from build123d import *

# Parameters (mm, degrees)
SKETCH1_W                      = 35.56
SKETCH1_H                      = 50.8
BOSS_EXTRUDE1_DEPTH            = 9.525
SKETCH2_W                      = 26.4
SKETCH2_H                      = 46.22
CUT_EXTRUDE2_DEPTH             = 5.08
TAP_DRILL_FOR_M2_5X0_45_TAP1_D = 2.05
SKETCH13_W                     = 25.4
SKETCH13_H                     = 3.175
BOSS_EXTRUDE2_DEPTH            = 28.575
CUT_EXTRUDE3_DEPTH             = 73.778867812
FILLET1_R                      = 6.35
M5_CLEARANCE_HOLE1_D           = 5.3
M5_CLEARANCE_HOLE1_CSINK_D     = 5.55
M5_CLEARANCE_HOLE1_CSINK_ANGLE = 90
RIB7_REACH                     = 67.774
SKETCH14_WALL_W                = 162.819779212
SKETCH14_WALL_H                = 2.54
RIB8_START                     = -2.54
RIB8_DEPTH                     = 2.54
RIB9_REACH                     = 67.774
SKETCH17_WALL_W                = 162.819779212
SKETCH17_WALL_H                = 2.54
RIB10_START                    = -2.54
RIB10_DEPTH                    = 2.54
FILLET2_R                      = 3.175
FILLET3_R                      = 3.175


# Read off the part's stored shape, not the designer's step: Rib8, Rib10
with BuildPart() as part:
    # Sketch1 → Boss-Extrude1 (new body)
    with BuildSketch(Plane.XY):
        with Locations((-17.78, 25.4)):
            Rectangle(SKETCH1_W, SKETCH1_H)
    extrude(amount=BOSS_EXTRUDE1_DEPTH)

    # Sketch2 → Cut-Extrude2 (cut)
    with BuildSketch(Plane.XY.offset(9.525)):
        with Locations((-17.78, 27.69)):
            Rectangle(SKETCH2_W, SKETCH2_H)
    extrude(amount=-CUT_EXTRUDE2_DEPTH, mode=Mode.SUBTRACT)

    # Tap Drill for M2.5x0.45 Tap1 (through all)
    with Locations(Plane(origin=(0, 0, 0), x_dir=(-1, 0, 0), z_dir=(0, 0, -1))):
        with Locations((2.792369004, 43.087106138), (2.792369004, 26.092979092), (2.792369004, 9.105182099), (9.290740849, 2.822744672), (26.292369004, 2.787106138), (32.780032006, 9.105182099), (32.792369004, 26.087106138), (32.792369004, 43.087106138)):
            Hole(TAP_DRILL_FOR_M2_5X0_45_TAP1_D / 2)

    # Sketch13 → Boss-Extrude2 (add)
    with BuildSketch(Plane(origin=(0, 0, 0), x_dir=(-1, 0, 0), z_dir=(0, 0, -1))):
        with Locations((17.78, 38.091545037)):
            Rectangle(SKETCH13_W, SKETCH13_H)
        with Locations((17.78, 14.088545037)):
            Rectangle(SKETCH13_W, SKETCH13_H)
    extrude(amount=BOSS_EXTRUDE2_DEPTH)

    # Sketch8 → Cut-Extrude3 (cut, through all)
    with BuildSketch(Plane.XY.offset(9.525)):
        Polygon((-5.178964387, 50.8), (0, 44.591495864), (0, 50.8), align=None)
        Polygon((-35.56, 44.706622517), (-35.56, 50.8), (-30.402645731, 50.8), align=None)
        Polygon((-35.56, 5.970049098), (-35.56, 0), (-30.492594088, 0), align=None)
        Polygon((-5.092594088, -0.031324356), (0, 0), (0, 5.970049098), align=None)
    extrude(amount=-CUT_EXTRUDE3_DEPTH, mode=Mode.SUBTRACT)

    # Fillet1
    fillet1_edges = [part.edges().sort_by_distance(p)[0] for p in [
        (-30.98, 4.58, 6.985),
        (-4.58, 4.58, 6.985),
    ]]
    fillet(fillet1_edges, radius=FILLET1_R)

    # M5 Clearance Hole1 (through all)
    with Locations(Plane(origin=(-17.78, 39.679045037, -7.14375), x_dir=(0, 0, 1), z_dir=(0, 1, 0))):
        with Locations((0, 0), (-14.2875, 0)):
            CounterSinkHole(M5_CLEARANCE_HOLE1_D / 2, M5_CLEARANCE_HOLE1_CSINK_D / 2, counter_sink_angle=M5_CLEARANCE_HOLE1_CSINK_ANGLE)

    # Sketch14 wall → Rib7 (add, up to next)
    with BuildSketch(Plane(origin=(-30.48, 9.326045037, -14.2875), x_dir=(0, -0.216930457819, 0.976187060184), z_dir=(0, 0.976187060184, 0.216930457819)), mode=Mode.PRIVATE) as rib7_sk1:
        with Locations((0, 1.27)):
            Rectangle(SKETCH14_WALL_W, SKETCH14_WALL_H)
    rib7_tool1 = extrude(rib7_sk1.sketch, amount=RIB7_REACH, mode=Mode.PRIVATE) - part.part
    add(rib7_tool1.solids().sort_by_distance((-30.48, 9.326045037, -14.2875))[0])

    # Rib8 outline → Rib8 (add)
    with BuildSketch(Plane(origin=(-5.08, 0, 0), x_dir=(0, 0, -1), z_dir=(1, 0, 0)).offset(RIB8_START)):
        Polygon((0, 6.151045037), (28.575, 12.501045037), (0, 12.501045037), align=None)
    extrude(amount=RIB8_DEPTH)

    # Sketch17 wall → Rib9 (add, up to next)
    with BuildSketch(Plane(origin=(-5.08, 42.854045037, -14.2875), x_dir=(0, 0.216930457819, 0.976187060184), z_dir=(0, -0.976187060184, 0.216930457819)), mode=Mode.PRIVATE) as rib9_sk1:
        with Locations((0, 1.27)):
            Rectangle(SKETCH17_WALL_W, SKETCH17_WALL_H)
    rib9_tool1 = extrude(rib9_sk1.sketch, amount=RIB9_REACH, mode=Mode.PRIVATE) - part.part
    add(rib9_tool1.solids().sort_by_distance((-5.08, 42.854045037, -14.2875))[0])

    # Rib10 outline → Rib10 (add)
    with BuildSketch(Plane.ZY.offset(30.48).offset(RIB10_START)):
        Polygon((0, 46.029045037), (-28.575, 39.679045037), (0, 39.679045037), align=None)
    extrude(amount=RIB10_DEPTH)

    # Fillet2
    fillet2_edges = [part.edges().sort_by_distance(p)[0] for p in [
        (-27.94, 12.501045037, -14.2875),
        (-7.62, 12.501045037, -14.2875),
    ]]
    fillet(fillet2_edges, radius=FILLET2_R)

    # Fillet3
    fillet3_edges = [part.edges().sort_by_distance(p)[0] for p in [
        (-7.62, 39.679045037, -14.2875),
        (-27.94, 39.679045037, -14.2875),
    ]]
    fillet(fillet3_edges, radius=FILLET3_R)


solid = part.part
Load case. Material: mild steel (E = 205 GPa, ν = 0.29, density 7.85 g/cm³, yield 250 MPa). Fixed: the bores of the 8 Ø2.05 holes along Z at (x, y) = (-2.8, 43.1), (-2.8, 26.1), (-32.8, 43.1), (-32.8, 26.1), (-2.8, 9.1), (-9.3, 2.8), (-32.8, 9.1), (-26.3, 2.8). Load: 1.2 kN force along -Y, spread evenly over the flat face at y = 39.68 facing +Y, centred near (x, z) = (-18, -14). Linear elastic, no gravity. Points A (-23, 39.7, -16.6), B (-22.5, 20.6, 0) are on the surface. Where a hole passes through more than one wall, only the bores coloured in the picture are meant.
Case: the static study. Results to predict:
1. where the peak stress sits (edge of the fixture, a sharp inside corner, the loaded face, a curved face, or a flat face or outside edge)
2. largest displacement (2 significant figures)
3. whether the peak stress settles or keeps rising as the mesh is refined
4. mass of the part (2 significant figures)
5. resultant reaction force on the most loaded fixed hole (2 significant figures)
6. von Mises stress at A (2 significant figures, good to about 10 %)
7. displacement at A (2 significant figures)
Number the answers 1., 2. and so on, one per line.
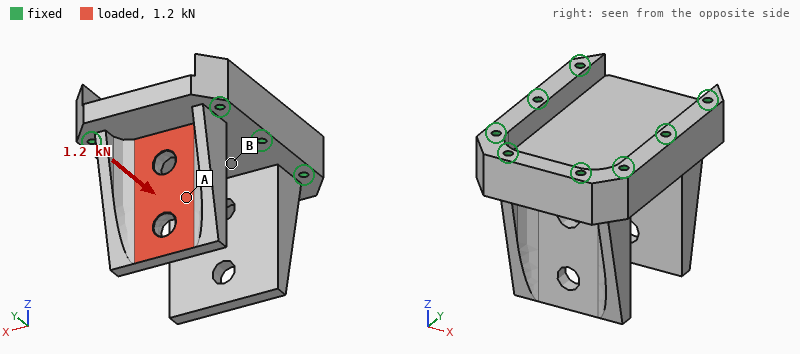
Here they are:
1. edge of the fixture
2. 79 µm
3. keeps rising
4. 120 g
5. 570 N
6. 39 MPa
7. 36 µm
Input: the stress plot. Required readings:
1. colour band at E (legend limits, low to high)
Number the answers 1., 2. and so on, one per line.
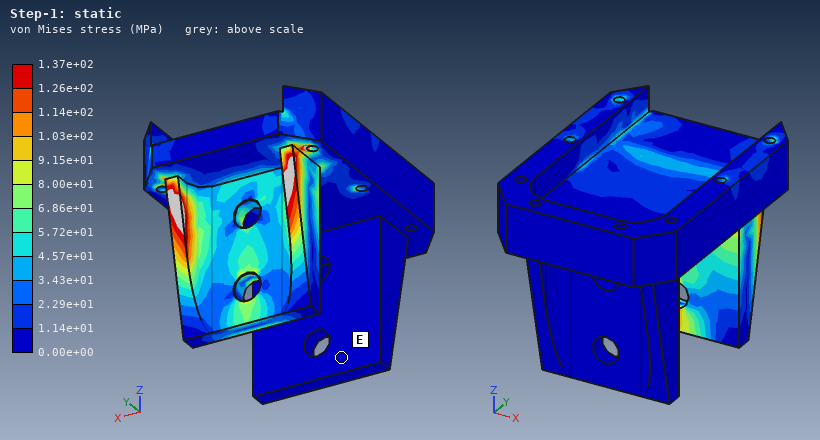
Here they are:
1. 0.00e+00 to 1.14e+01 MPa
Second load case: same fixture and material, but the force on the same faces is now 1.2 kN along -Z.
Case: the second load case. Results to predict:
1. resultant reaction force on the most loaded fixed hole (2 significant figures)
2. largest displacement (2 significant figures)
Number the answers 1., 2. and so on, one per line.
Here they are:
1. 490 N
2. 4.5 µm
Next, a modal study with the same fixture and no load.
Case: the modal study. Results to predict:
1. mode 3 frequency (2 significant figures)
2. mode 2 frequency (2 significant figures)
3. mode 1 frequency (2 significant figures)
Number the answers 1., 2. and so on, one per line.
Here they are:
1. 10 kHz
2. 6100 Hz
3. 5900 Hz
